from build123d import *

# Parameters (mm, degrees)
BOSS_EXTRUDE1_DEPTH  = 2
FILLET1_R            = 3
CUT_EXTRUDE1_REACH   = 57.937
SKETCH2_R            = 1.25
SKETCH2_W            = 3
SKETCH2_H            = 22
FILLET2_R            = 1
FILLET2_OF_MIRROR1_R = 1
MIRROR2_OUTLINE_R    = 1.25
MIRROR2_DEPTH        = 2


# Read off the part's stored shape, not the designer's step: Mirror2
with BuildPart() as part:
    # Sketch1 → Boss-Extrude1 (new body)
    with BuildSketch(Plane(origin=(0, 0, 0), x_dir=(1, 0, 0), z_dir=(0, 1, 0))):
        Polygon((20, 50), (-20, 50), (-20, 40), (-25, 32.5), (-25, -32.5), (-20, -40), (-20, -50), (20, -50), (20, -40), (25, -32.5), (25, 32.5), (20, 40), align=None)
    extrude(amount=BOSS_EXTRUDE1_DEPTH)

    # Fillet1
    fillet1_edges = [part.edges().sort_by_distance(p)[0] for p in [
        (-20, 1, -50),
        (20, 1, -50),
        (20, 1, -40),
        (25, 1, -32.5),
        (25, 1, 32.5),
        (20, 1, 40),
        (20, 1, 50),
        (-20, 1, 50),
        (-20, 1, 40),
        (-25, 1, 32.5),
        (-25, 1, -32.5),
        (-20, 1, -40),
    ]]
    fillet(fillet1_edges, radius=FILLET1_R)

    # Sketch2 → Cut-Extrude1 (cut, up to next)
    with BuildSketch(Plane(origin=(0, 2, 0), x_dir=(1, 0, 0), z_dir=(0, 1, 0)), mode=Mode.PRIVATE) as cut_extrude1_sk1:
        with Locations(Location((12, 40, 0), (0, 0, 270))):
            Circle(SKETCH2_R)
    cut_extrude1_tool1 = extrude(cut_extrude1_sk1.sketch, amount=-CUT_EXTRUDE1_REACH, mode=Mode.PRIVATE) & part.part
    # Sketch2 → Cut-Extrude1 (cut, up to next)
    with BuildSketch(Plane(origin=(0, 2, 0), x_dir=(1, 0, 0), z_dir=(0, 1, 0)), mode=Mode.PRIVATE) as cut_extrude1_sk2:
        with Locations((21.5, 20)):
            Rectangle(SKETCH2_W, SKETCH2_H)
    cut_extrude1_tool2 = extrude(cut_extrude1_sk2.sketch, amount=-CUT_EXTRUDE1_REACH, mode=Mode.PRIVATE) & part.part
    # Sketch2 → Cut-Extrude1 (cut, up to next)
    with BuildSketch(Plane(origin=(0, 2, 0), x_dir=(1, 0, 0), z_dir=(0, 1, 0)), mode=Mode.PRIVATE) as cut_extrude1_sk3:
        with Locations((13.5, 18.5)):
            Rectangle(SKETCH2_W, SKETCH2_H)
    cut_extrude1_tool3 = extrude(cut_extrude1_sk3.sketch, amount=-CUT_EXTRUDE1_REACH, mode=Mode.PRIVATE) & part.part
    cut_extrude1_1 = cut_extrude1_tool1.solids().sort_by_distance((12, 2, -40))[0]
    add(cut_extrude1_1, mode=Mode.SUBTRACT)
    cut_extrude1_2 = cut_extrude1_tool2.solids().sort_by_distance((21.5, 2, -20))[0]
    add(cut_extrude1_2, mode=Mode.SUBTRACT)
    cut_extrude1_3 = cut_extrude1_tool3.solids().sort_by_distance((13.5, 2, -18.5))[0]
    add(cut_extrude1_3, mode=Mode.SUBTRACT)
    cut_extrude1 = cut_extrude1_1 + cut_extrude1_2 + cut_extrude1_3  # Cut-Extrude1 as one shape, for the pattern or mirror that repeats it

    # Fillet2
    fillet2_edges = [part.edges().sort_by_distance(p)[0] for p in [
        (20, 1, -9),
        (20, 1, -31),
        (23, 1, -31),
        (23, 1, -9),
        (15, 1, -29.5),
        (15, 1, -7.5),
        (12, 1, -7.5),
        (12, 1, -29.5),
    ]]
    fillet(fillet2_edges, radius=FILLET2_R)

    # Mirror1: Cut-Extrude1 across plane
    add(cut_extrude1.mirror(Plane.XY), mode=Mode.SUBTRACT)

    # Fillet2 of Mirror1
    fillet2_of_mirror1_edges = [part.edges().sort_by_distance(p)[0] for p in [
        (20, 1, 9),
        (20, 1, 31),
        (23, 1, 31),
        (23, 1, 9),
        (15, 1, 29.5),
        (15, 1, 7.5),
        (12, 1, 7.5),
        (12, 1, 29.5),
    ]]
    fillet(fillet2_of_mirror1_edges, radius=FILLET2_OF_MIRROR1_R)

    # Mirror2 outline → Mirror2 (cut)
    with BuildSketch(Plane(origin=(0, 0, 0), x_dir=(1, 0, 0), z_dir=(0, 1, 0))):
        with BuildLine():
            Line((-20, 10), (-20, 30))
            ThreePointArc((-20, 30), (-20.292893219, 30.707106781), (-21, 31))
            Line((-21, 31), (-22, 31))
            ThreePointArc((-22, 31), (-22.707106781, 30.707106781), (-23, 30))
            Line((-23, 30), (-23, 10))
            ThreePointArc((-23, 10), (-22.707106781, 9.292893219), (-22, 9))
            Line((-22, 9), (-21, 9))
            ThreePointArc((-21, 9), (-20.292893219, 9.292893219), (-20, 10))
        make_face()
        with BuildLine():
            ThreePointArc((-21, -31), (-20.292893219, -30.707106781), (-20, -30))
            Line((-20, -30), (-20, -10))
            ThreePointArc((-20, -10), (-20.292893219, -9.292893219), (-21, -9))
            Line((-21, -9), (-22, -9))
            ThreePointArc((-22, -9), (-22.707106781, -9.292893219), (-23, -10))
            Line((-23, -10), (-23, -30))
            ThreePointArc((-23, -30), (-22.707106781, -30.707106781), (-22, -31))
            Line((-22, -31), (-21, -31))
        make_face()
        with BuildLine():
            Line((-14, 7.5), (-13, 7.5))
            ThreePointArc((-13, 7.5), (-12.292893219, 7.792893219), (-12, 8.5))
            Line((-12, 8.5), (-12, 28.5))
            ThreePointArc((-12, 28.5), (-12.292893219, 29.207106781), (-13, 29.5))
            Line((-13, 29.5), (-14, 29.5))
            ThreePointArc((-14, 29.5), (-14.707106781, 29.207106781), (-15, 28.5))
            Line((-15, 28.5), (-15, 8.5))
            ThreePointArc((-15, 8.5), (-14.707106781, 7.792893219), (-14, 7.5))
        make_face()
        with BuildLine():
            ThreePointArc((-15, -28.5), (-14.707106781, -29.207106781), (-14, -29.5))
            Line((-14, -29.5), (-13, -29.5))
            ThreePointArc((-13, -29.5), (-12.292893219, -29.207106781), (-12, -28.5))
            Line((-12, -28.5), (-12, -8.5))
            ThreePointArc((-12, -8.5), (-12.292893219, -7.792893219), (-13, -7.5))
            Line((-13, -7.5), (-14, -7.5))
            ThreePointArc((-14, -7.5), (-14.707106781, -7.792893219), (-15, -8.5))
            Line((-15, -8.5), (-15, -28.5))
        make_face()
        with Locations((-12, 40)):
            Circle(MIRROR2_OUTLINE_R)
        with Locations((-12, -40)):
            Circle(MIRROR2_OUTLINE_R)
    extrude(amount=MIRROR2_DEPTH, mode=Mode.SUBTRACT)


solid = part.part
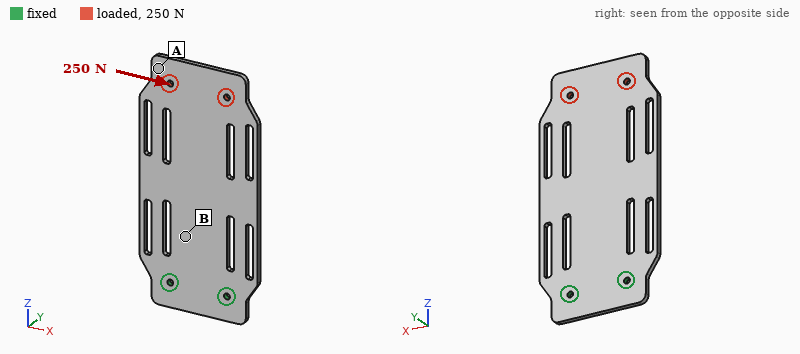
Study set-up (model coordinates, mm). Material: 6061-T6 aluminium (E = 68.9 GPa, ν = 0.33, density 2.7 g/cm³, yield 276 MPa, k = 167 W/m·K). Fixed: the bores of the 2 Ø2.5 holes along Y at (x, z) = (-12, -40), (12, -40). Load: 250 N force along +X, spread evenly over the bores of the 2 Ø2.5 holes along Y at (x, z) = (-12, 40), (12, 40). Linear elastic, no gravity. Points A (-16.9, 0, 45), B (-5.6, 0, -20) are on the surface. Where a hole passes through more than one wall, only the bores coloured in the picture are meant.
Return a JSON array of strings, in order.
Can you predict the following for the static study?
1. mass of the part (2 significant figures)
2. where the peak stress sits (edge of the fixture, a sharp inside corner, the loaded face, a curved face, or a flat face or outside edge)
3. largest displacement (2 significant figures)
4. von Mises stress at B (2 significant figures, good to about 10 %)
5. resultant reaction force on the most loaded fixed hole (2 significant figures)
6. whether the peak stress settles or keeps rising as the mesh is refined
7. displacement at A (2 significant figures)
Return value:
["23 g", "edge of the fixture", "97 µm", "14 MPa", "810 N", "keeps rising", "92 µm"]
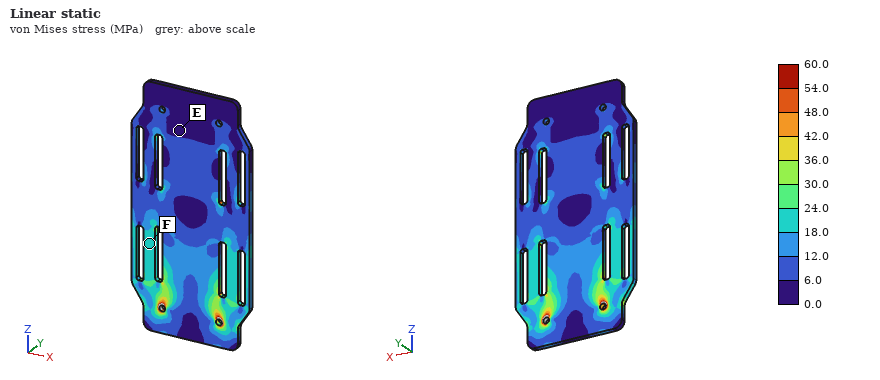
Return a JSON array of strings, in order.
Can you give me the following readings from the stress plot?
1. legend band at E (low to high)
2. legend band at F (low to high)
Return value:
["0.0 to 6.0 MPa", "18.0 to 24.0 MPa"]
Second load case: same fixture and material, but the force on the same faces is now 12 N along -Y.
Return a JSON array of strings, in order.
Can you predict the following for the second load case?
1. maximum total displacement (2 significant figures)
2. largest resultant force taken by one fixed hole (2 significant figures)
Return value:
["1.3 mm", "6.0 N"]
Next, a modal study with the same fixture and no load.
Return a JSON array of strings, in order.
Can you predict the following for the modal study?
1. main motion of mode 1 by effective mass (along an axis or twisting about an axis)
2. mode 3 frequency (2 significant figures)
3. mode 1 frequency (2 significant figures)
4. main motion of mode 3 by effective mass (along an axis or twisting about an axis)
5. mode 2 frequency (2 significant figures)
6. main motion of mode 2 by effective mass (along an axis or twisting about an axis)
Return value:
["along Y", "1200 Hz", "200 Hz", "along Y", "820 Hz", "twisting about Z"]
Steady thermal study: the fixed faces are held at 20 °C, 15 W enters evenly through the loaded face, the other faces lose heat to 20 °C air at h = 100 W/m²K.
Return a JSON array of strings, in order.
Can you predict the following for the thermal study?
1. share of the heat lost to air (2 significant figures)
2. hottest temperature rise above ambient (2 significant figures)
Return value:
["83 %", "37 K"]
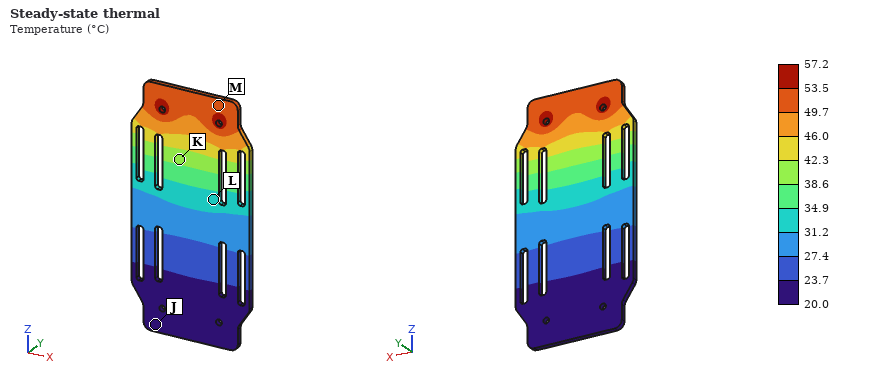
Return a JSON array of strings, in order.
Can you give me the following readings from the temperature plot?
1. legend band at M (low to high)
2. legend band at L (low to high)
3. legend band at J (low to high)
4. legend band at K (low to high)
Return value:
["49.7 to 53.5 °C", "31.2 to 34.9 °C", "20.0 to 23.7 °C", "38.6 to 42.3 °C"]
